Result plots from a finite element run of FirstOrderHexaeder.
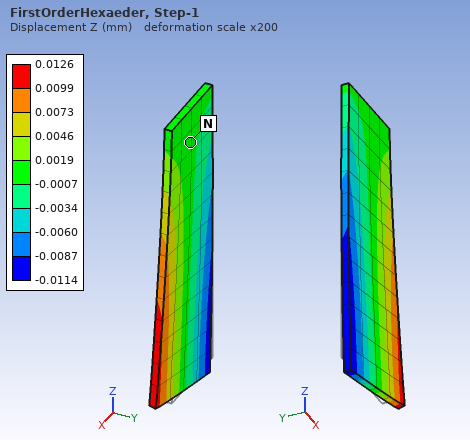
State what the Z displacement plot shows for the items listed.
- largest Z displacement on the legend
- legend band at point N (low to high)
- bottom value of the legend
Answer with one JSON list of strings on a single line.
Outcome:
["0.0126 mm", "-0.0007 to 0.0019 mm", "-0.0114 mm"]
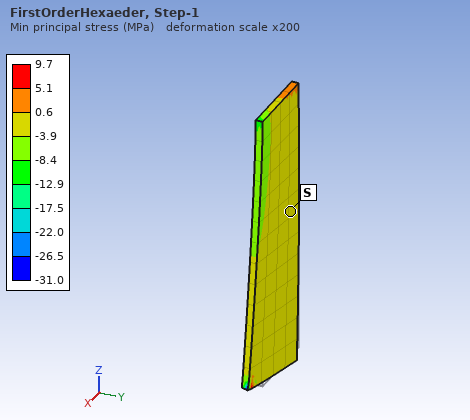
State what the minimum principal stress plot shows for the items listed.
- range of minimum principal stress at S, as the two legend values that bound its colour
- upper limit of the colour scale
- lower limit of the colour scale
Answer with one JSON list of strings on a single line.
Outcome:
["-3.9 to 0.6 MPa", "9.7 MPa", "-31.0 MPa"]
